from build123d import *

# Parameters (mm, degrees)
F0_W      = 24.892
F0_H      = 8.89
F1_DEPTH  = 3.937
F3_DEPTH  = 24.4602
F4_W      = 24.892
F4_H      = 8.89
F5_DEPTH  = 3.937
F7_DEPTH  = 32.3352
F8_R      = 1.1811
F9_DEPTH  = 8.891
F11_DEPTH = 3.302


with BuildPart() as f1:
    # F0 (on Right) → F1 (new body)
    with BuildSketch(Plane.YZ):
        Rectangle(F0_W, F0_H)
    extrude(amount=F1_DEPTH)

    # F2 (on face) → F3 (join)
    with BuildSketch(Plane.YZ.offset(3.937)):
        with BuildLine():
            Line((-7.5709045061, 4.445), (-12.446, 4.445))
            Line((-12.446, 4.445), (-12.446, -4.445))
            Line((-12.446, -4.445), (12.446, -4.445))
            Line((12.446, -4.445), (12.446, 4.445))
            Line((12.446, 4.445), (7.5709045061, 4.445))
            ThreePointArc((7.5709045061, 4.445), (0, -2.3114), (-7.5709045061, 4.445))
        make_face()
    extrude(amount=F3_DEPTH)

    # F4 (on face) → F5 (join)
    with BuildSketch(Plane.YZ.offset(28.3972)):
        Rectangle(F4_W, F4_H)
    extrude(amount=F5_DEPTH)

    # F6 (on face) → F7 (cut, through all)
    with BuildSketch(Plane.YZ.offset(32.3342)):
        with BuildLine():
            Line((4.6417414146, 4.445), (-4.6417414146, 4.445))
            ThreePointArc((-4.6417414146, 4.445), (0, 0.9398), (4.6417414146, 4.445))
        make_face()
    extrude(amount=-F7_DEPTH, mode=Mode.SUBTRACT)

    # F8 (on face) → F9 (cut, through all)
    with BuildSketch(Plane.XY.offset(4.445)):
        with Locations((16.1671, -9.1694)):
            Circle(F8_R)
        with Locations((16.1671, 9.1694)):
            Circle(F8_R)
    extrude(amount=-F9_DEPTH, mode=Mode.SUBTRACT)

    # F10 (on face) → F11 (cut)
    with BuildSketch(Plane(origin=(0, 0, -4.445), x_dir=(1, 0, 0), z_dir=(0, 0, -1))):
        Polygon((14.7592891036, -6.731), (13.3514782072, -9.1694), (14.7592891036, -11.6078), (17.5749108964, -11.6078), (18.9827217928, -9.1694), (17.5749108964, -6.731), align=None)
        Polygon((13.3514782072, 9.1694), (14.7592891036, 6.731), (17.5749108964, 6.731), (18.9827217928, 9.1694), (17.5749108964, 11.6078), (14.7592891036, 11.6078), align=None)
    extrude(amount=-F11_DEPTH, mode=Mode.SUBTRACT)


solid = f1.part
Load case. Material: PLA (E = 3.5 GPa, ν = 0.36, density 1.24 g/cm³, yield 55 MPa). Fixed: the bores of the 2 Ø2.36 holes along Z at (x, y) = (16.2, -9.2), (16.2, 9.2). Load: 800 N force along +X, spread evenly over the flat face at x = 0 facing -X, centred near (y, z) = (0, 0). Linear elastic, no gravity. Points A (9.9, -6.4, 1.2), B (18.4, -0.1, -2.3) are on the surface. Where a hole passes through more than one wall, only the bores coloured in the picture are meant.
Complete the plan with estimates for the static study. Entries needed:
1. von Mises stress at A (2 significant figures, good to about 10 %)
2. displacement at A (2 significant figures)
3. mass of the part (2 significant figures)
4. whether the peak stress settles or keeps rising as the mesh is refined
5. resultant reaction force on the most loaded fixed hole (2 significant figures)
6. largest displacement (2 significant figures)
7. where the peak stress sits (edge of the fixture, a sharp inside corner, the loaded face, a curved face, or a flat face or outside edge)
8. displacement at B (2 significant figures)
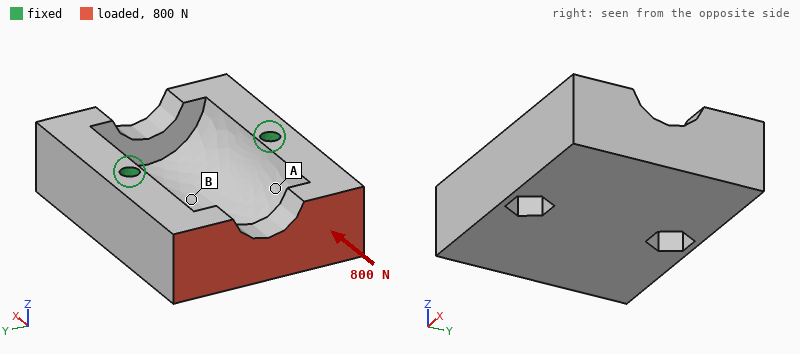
9.5 MPa
29 µm
6.0 g
keeps rising
400 N
78 µm
edge of the fixture
26 µm
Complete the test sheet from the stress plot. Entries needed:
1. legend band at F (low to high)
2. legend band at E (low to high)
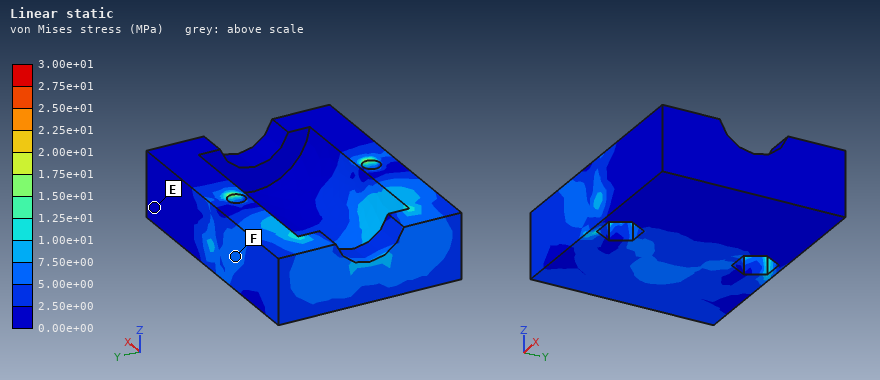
5.00e+00 to 7.50e+00 MPa
0.00e+00 to 2.50e+00 MPa
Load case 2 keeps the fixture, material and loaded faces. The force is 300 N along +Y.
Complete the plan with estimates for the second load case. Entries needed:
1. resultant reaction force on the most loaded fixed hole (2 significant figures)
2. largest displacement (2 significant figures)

270 N
0.16 mm
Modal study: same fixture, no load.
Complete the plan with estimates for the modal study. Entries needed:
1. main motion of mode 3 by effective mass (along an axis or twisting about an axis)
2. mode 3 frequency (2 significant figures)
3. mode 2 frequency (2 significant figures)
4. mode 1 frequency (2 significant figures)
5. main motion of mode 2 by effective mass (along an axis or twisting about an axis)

along Z
6000 Hz
5500 Hz
3700 Hz
twisting about Z
